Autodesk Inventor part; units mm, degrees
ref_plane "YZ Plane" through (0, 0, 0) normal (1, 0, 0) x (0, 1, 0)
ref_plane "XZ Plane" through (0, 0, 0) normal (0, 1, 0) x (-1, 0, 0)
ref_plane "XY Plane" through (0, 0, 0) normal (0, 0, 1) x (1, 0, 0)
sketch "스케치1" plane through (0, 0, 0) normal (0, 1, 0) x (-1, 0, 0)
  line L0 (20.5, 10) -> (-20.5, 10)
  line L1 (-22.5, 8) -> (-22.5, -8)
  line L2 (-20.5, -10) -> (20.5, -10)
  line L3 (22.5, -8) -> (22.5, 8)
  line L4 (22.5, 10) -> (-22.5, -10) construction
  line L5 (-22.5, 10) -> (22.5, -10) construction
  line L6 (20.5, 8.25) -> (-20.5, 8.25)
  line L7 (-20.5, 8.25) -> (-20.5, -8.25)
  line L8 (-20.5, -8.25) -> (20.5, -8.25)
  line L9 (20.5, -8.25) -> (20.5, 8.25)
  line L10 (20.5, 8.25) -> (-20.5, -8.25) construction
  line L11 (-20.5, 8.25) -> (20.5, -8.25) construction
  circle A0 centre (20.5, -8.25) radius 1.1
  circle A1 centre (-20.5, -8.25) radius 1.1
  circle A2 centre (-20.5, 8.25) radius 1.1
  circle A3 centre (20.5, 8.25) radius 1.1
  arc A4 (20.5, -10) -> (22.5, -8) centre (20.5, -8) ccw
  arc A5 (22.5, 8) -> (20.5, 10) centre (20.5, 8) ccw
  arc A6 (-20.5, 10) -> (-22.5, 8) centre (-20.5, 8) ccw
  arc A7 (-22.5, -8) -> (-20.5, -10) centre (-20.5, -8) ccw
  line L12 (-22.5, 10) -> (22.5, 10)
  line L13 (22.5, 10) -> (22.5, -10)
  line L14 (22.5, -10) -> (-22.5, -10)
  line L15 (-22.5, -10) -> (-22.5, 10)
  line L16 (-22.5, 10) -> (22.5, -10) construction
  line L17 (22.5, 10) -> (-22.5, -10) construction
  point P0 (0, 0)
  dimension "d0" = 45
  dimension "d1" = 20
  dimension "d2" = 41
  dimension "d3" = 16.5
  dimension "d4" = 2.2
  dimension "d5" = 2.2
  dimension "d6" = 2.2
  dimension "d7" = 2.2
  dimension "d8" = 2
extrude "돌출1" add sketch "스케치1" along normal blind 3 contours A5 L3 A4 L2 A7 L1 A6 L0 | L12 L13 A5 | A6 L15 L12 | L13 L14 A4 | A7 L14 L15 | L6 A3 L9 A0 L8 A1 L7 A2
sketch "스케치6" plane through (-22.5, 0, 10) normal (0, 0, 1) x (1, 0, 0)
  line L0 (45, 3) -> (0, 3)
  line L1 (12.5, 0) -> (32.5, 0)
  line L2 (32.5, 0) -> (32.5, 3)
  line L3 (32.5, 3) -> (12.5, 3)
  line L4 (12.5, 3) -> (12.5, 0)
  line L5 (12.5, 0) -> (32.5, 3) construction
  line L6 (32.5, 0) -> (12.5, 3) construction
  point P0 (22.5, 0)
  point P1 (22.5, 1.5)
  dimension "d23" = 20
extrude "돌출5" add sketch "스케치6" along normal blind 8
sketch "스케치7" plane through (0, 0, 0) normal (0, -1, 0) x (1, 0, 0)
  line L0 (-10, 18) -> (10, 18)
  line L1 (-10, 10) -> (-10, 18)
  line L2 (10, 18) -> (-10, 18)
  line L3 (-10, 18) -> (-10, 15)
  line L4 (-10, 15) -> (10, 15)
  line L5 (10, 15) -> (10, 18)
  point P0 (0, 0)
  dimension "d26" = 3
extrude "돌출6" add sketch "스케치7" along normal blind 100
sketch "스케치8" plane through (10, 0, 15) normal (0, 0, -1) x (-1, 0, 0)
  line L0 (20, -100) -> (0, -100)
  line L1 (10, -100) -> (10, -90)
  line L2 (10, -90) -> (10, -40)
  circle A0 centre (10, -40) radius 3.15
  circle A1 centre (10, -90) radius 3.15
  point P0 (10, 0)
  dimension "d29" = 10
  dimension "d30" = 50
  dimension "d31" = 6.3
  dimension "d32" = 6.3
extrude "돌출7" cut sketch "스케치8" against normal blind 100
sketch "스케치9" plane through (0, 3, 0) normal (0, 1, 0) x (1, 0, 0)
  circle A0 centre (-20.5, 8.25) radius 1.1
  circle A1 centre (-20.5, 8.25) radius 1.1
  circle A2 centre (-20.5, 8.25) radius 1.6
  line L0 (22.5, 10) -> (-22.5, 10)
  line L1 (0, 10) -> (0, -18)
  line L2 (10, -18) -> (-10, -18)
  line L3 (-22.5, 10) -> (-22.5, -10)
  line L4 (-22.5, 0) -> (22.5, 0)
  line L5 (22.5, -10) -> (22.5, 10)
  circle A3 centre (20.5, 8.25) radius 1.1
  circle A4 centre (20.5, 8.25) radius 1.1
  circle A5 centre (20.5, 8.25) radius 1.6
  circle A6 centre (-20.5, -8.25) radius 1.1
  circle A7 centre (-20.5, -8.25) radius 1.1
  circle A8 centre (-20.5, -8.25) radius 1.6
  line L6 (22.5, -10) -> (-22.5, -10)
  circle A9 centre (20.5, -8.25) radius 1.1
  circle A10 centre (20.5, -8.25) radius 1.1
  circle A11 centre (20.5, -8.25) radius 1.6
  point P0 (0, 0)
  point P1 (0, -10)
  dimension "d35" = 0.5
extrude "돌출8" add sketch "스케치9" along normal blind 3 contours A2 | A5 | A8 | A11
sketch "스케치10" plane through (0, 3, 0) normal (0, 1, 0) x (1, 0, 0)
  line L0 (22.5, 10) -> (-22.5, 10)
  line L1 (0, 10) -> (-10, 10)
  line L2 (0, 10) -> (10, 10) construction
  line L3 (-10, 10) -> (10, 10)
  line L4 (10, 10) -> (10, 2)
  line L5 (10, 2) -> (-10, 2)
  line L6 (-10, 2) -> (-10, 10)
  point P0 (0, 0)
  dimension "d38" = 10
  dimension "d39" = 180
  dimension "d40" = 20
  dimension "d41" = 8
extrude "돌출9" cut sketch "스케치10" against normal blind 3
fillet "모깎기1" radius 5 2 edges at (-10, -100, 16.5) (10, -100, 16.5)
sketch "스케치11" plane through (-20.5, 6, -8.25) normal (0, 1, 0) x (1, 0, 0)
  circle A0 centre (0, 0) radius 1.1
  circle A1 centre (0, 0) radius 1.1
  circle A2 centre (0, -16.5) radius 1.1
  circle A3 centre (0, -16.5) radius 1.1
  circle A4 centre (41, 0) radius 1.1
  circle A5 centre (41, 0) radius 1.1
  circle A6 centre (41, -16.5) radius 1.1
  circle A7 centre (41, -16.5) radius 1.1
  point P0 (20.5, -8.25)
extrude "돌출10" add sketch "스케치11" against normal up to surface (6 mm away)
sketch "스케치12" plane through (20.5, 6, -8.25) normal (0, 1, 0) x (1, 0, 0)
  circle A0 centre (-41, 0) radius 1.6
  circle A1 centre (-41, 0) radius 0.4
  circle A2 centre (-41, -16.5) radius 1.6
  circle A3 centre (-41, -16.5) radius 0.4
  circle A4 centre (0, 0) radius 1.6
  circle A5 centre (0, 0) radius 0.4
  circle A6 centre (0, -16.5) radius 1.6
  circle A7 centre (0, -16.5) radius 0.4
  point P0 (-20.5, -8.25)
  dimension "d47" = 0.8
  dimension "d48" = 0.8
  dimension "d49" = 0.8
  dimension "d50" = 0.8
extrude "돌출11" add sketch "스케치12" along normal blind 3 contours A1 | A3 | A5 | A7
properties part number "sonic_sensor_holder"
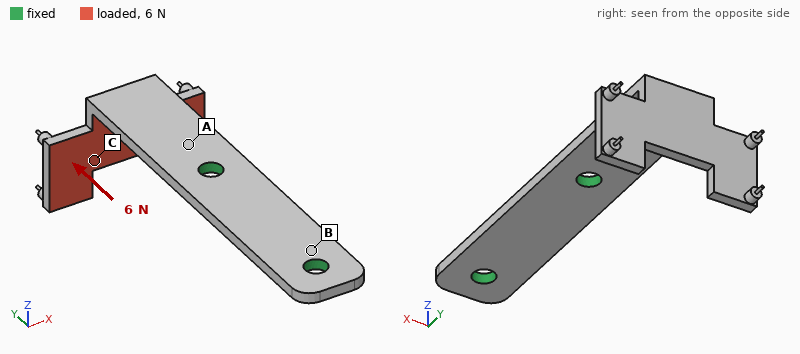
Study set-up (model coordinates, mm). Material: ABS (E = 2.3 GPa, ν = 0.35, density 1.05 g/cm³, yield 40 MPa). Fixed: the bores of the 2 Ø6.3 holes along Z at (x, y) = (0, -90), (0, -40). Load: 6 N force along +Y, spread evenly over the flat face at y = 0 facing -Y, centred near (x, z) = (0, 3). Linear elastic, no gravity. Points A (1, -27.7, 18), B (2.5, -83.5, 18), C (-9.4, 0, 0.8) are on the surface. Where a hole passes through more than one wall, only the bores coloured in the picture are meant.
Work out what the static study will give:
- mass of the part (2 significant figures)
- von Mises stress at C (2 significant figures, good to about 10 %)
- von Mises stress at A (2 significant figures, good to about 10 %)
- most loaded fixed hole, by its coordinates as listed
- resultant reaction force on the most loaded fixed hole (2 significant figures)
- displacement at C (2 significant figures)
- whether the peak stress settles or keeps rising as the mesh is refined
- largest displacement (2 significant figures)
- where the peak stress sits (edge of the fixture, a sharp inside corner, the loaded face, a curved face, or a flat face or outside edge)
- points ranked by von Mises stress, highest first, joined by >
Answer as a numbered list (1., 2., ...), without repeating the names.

1. 9.0 g
2. 0.59 MPa
3. 2.5 MPa
4. (0, -40)
5. 5.7 N
6. 0.78 mm
7. keeps rising
8. 1.3 mm
9. edge of the fixture
10. A > C > B
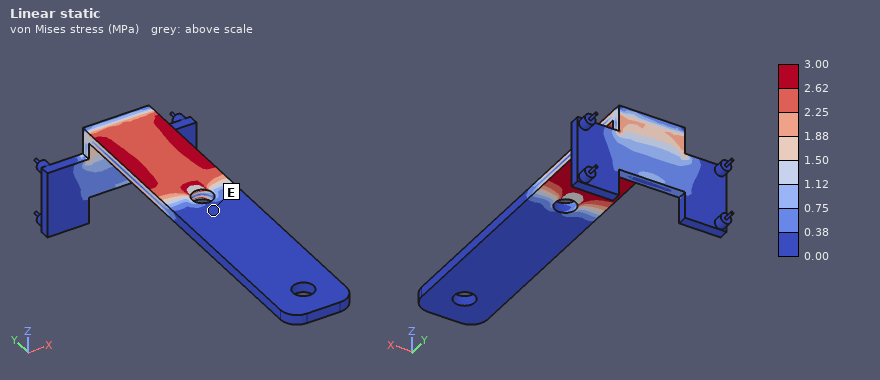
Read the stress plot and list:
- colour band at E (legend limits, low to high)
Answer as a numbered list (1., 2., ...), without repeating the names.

1. 0.00 to 0.38 MPa
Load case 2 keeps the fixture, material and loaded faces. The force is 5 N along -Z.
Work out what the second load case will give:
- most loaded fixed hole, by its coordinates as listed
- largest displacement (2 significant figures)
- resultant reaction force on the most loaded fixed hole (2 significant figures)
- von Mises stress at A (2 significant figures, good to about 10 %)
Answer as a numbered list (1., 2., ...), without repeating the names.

1. (0, -40)
2. 1.4 mm
3. 5.0 N
4. 4.2 MPa
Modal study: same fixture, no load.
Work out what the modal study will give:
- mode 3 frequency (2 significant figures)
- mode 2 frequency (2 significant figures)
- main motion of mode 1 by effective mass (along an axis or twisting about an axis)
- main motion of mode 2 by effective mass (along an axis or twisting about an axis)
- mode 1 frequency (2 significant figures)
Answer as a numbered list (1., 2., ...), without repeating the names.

1. 570 Hz
2. 280 Hz
3. along Z
4. along X
5. 170 Hz
